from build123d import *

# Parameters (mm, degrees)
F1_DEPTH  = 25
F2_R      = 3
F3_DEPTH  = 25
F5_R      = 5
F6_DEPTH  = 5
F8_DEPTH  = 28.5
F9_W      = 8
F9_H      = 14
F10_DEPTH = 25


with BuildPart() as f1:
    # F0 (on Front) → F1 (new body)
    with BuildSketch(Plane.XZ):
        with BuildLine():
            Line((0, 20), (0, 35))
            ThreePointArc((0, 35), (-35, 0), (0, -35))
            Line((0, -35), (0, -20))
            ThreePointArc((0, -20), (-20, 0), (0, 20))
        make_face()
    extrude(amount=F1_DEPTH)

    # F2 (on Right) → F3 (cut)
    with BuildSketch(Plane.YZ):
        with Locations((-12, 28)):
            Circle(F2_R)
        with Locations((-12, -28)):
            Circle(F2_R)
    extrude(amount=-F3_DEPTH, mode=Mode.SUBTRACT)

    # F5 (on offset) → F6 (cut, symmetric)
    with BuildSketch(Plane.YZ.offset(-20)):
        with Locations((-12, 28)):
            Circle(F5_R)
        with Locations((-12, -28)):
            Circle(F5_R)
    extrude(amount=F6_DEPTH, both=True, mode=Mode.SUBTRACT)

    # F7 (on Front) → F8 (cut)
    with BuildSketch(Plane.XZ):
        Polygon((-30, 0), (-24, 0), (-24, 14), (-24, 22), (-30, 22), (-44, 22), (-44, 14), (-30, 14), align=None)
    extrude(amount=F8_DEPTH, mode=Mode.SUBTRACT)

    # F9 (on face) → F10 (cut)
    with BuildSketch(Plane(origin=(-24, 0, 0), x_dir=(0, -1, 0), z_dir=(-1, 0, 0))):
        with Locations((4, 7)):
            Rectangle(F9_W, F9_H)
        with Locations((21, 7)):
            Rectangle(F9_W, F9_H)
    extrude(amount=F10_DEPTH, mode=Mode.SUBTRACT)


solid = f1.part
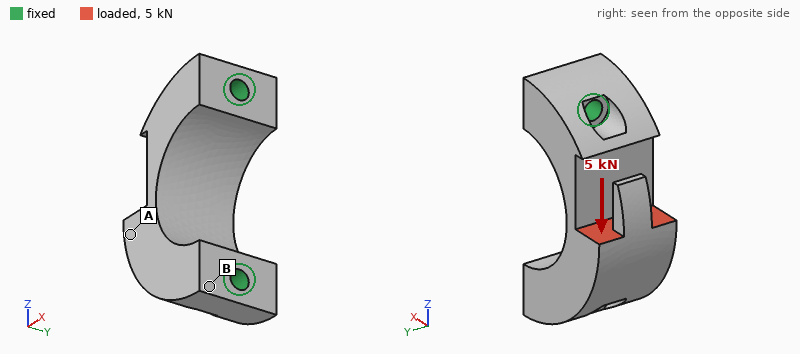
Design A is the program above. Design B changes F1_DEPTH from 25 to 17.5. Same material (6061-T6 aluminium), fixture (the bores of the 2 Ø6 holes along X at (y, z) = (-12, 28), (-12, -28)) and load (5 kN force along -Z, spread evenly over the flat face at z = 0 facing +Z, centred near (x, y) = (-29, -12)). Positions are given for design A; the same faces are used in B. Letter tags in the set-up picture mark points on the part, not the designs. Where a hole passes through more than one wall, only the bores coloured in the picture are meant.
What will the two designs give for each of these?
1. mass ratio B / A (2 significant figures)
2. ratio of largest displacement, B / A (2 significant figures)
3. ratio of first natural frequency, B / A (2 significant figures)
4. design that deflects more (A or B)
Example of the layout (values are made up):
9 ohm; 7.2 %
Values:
0.69; 1.4; 0.92; B
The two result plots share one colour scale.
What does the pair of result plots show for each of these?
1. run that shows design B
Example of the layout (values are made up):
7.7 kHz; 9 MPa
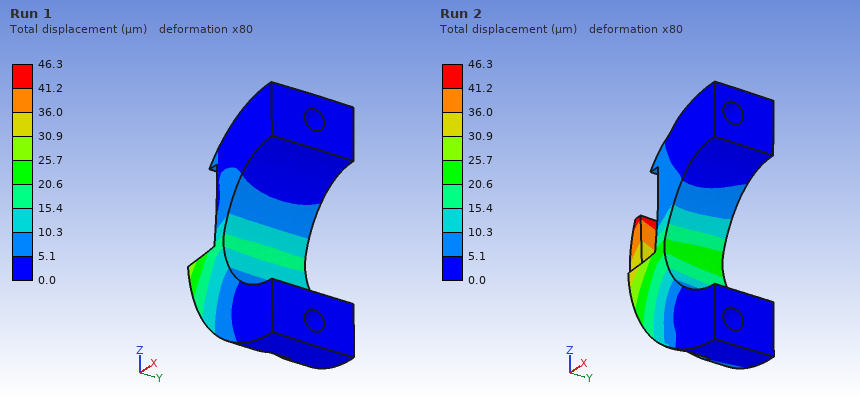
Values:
Run 2
